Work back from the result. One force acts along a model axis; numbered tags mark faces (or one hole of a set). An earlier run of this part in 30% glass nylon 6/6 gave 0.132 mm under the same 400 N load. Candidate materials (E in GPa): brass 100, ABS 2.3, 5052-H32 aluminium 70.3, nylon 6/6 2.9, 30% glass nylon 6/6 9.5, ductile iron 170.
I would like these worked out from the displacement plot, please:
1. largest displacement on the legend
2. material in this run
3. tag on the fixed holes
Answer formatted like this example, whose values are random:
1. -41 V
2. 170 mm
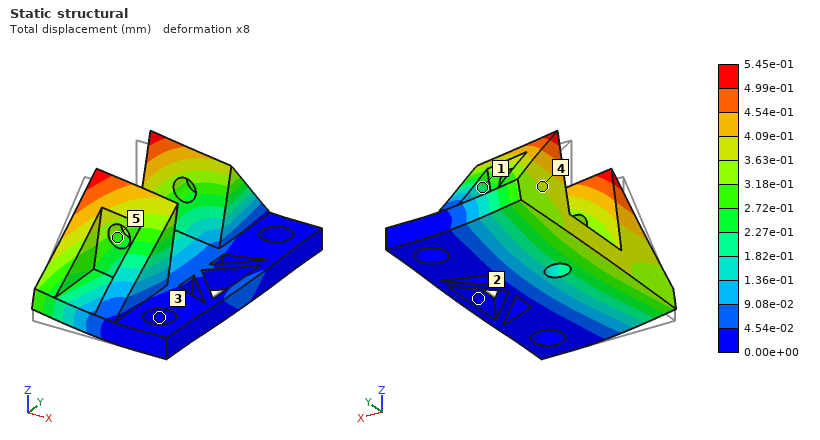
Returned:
1. 5.45e-01 mm
2. ABS
3. 3
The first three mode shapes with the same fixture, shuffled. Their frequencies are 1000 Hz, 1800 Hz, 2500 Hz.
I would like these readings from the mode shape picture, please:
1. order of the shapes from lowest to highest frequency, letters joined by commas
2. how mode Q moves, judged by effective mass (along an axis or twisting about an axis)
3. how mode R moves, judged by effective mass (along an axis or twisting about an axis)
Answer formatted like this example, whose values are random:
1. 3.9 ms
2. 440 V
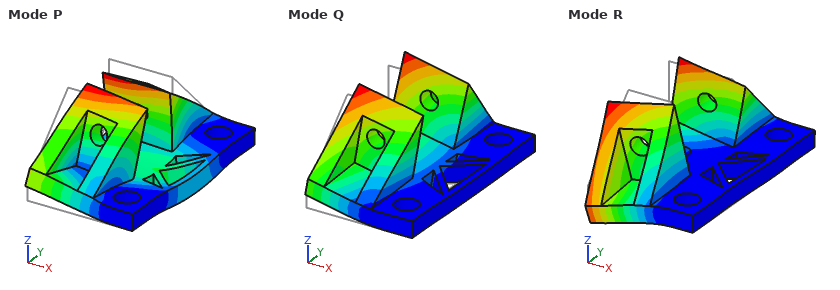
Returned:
1. Q, R, P
2. along Z
3. twisting about X
